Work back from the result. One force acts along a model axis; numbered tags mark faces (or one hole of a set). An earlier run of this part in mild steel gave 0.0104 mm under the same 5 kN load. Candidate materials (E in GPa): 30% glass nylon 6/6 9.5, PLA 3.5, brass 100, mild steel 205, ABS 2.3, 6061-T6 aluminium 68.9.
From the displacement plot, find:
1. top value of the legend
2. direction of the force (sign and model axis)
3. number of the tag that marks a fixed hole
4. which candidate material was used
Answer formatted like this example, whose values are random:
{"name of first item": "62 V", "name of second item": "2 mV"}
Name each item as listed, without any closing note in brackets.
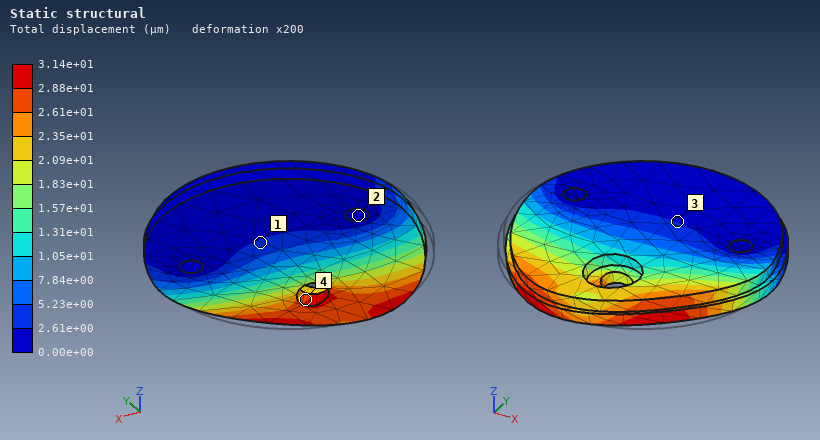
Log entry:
{"top value of the legend": "3.14e+01 µm", "direction of the force": "+X", "number of the tag that marks a fixed hole": "2", "which candidate material was used": "6061-T6 aluminium"}
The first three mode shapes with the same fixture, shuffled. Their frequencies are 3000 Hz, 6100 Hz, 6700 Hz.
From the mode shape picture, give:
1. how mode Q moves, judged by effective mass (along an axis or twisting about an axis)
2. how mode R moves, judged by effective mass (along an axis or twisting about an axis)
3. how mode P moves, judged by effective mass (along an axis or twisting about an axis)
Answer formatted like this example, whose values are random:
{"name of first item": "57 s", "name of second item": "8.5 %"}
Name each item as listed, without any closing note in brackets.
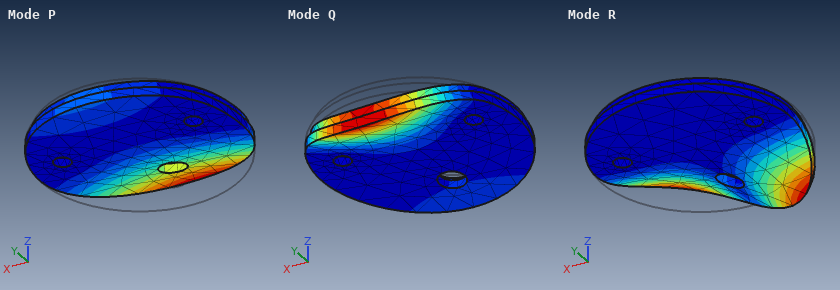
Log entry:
{"how mode Q moves, judged by effective mass": "along Z", "how mode R moves, judged by effective mass": "twisting about Y", "how mode P moves, judged by effective mass": "along Z"}
